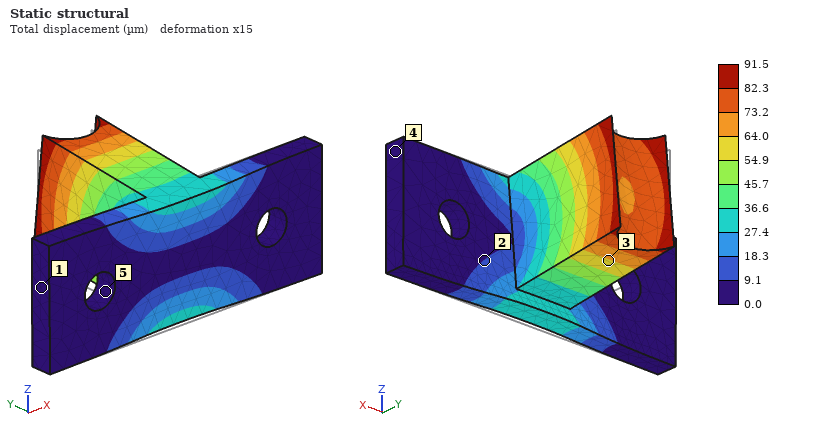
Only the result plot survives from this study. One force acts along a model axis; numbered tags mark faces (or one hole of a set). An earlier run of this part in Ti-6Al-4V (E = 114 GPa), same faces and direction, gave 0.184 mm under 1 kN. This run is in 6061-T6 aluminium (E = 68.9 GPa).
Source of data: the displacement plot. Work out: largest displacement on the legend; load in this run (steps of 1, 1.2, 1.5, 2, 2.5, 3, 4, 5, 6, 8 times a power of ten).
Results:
91.5 µm
300 N
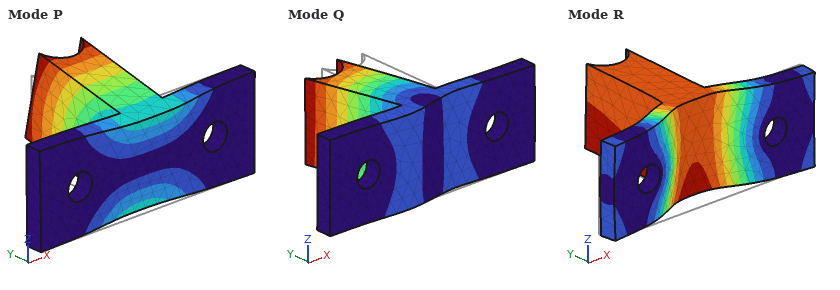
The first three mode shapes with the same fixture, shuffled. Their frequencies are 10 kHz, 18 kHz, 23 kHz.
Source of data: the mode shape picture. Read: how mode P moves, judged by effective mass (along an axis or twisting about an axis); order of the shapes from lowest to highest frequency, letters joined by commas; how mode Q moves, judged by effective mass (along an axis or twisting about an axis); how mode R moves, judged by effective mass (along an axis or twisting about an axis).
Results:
along Z
P, Q, R
along X
along Y
